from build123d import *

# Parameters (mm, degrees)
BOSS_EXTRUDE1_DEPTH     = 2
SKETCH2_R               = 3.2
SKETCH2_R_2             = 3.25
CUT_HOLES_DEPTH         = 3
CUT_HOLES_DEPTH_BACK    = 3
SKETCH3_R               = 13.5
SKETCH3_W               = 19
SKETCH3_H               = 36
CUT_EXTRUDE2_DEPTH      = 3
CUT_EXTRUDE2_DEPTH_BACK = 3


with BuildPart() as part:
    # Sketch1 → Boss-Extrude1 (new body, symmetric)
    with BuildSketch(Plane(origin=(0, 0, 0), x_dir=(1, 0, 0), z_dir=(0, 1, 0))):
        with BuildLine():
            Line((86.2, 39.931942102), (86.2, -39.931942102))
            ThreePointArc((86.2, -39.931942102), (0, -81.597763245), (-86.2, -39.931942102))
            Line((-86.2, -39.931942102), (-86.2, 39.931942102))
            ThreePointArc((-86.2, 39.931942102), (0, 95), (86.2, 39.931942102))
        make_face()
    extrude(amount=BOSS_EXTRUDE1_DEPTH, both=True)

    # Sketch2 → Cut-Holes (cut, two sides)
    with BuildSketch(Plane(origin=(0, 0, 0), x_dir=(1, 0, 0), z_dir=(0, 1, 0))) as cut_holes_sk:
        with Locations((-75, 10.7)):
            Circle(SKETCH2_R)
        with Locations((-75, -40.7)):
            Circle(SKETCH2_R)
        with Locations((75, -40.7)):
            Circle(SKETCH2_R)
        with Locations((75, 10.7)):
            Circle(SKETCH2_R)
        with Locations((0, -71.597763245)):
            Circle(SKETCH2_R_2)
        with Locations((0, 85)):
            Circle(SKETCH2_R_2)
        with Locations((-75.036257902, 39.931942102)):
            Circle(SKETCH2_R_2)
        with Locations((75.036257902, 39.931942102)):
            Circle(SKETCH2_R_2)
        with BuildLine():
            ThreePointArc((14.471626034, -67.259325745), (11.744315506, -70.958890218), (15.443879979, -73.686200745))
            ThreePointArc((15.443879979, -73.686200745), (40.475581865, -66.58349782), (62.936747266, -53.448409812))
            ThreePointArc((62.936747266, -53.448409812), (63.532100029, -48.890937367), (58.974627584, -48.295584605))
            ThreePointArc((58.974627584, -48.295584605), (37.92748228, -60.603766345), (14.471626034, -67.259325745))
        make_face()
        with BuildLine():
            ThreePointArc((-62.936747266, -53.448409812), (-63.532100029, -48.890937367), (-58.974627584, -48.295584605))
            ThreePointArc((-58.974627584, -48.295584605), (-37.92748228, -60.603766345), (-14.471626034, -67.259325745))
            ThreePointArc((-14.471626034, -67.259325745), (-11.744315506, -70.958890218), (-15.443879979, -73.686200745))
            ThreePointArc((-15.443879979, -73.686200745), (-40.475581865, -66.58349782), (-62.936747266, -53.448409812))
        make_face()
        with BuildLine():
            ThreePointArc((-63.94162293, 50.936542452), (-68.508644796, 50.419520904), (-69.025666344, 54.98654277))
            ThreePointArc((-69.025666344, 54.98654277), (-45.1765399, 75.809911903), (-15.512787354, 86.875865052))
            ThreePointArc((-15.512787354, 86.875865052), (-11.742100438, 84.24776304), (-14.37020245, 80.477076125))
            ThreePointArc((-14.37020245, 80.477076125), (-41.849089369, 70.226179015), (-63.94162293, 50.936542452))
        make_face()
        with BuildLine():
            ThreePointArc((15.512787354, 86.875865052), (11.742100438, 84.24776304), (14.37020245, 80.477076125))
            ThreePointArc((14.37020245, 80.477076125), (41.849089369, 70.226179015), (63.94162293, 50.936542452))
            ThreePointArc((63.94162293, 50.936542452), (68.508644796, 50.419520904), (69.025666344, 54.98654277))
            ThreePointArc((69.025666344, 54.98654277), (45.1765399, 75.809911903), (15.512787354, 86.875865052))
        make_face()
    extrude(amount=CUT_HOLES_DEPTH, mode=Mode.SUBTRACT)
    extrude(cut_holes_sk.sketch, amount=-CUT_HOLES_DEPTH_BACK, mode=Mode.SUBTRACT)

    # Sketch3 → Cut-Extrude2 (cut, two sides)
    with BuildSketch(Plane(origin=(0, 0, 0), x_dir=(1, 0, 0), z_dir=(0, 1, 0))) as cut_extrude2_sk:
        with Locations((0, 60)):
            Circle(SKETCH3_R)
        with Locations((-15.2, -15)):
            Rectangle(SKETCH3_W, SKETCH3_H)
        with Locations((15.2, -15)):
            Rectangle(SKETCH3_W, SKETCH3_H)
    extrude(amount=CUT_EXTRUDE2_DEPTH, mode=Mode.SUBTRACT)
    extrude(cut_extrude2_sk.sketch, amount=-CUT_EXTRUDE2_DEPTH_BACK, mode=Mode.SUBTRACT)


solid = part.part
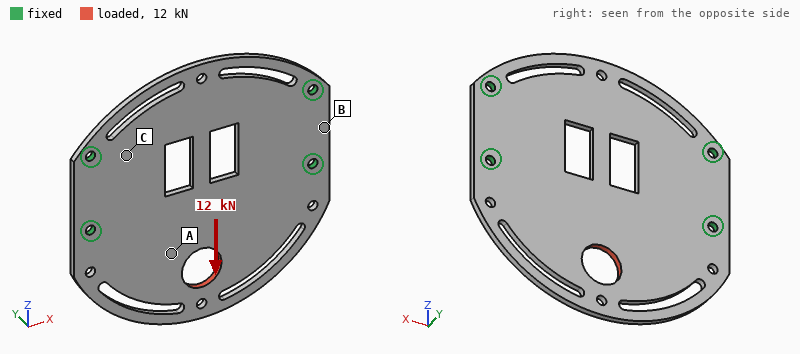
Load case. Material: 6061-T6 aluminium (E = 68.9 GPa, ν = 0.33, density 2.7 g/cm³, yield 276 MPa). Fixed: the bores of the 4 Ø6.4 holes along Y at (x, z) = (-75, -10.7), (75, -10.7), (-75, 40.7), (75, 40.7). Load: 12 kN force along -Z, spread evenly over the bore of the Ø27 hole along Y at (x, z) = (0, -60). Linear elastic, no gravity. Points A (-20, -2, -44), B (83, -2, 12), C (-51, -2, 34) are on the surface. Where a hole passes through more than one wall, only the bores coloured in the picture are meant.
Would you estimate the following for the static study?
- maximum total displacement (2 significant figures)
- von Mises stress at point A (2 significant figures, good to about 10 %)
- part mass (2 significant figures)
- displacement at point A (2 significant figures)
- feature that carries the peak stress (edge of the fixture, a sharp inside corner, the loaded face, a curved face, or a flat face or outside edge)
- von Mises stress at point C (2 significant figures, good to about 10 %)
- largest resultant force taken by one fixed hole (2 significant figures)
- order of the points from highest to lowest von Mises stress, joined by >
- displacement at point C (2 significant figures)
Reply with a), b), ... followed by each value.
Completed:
a) 79 µm
b) 35 MPa
c) 240 g
d) 49 µm
e) a curved face
f) 21 MPa
g) 3.9 kN
h) A > C > B
i) 15 µm
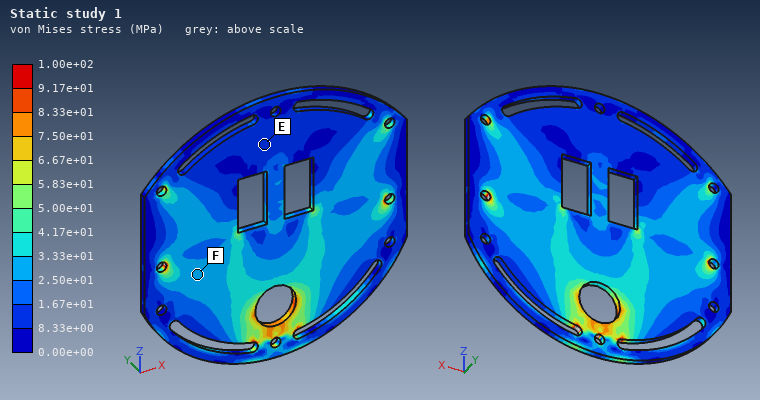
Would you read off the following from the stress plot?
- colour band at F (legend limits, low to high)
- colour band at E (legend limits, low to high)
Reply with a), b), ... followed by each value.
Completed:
a) 2.50e+01 to 3.33e+01 MPa
b) 8.33e+00 to 1.67e+01 MPa
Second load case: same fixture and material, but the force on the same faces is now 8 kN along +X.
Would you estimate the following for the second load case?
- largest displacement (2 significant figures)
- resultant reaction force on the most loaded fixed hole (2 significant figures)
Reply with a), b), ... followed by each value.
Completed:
a) 63 µm
b) 4.2 kN
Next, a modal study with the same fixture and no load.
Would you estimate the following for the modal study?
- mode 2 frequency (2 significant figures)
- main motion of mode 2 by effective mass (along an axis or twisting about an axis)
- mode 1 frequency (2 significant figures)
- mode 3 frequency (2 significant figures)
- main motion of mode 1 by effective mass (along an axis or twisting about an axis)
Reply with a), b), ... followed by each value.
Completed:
a) 810 Hz
b) along Y
c) 460 Hz
d) 1100 Hz
e) along Y
